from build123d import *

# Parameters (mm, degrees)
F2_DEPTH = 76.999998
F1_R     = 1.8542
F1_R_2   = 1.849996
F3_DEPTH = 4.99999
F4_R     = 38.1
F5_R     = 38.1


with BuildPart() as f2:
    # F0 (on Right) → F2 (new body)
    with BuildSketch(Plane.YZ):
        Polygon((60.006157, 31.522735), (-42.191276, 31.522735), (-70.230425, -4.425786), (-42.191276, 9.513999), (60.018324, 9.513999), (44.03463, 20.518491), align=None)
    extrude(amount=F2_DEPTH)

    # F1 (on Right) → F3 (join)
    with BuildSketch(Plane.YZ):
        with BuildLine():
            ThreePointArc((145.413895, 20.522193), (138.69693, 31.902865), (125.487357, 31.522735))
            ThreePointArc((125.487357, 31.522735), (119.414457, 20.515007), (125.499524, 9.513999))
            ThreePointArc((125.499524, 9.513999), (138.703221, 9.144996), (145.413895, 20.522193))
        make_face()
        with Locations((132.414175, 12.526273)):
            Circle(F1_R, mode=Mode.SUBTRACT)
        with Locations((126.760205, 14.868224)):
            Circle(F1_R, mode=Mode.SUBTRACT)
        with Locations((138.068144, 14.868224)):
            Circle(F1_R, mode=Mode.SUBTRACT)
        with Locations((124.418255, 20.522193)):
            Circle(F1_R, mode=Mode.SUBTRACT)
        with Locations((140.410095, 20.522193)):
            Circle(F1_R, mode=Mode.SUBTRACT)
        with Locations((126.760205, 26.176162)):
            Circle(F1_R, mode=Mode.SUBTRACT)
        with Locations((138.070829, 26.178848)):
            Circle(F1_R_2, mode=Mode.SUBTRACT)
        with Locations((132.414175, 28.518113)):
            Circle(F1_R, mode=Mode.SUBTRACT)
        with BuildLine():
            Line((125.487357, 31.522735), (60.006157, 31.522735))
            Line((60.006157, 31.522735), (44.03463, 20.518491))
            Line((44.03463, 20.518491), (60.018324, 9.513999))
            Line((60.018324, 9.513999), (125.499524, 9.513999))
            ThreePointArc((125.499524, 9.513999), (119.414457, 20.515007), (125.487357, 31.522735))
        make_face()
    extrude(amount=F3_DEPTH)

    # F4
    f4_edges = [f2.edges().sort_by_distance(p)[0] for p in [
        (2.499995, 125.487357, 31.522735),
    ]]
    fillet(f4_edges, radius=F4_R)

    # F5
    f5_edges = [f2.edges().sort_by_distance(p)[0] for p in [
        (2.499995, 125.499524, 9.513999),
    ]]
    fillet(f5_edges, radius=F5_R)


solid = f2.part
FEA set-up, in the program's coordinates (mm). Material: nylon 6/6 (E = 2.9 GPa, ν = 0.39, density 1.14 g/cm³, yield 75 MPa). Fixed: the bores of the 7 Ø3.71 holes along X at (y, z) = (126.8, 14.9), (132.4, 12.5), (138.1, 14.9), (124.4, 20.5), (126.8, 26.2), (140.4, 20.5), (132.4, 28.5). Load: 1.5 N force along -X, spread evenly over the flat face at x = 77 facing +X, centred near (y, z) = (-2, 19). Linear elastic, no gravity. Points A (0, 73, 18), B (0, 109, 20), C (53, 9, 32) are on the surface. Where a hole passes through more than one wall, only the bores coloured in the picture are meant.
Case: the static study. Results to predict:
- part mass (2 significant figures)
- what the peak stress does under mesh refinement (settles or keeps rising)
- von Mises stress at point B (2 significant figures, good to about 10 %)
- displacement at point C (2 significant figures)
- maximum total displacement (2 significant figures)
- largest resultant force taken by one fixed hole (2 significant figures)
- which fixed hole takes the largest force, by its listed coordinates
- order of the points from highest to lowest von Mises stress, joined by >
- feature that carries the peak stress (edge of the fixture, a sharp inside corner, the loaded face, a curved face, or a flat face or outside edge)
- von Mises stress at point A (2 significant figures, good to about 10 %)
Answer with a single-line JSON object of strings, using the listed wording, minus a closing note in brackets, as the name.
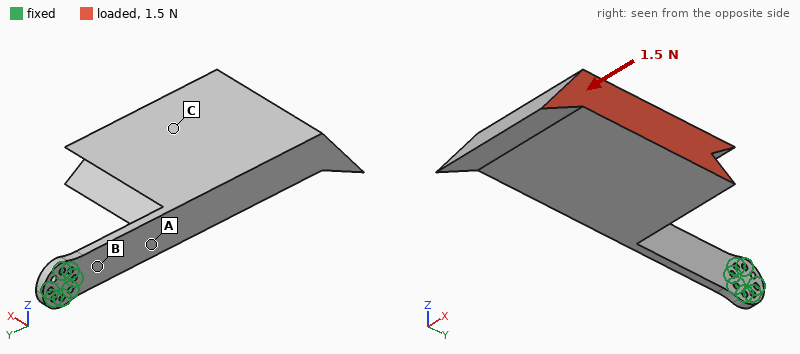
{"part mass": "220 g", "what the peak stress does under mesh refinement": "keeps rising", "von Mises stress at point B": "1.7 MPa", "displacement at point C": "1.4 mm", "maximum total displacement": "2.6 mm", "largest resultant force taken by one fixed hole": "11 N", "which fixed hole takes the largest force, by its listed coordinates": "(124.4, 20.5)", "order of the points from highest to lowest von Mises stress, joined by >": "B > A > C", "feature that carries the peak stress": "edge of the fixture", "von Mises stress at point A": "1.2 MPa"}
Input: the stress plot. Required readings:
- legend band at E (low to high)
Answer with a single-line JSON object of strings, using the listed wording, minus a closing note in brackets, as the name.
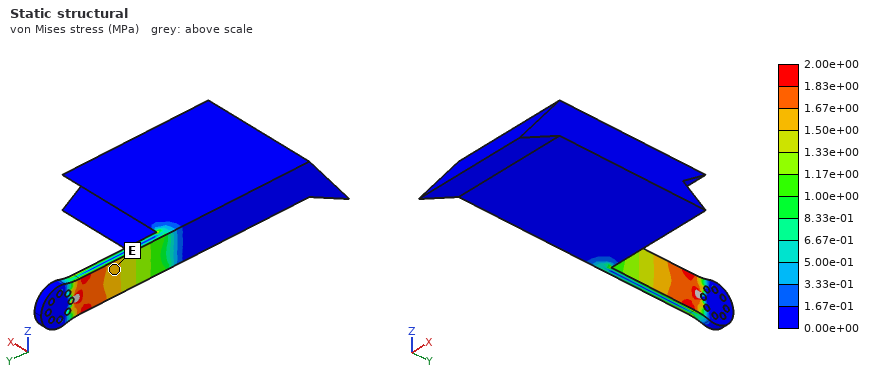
{"legend band at E": "1.50e+00 to 1.67e+00 MPa"}
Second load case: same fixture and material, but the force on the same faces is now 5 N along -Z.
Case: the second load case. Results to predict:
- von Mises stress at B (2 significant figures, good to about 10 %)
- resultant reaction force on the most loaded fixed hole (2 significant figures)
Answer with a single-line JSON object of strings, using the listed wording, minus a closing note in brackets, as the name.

{"von Mises stress at B": "3.8 MPa", "resultant reaction force on the most loaded fixed hole": "35 N"}
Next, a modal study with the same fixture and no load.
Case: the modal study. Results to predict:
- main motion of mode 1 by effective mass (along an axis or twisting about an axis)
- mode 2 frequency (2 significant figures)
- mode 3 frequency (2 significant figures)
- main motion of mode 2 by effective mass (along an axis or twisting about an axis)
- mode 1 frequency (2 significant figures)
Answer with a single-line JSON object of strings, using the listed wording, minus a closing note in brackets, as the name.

{"main motion of mode 1 by effective mass": "along X", "mode 2 frequency": "26 Hz", "mode 3 frequency": "83 Hz", "main motion of mode 2 by effective mass": "along Z", "mode 1 frequency": "10 Hz"}
